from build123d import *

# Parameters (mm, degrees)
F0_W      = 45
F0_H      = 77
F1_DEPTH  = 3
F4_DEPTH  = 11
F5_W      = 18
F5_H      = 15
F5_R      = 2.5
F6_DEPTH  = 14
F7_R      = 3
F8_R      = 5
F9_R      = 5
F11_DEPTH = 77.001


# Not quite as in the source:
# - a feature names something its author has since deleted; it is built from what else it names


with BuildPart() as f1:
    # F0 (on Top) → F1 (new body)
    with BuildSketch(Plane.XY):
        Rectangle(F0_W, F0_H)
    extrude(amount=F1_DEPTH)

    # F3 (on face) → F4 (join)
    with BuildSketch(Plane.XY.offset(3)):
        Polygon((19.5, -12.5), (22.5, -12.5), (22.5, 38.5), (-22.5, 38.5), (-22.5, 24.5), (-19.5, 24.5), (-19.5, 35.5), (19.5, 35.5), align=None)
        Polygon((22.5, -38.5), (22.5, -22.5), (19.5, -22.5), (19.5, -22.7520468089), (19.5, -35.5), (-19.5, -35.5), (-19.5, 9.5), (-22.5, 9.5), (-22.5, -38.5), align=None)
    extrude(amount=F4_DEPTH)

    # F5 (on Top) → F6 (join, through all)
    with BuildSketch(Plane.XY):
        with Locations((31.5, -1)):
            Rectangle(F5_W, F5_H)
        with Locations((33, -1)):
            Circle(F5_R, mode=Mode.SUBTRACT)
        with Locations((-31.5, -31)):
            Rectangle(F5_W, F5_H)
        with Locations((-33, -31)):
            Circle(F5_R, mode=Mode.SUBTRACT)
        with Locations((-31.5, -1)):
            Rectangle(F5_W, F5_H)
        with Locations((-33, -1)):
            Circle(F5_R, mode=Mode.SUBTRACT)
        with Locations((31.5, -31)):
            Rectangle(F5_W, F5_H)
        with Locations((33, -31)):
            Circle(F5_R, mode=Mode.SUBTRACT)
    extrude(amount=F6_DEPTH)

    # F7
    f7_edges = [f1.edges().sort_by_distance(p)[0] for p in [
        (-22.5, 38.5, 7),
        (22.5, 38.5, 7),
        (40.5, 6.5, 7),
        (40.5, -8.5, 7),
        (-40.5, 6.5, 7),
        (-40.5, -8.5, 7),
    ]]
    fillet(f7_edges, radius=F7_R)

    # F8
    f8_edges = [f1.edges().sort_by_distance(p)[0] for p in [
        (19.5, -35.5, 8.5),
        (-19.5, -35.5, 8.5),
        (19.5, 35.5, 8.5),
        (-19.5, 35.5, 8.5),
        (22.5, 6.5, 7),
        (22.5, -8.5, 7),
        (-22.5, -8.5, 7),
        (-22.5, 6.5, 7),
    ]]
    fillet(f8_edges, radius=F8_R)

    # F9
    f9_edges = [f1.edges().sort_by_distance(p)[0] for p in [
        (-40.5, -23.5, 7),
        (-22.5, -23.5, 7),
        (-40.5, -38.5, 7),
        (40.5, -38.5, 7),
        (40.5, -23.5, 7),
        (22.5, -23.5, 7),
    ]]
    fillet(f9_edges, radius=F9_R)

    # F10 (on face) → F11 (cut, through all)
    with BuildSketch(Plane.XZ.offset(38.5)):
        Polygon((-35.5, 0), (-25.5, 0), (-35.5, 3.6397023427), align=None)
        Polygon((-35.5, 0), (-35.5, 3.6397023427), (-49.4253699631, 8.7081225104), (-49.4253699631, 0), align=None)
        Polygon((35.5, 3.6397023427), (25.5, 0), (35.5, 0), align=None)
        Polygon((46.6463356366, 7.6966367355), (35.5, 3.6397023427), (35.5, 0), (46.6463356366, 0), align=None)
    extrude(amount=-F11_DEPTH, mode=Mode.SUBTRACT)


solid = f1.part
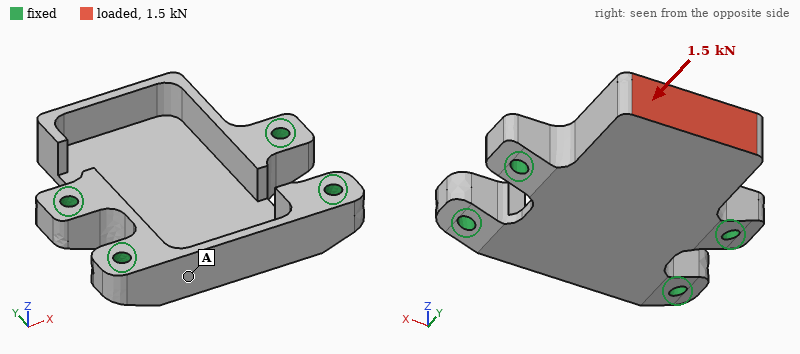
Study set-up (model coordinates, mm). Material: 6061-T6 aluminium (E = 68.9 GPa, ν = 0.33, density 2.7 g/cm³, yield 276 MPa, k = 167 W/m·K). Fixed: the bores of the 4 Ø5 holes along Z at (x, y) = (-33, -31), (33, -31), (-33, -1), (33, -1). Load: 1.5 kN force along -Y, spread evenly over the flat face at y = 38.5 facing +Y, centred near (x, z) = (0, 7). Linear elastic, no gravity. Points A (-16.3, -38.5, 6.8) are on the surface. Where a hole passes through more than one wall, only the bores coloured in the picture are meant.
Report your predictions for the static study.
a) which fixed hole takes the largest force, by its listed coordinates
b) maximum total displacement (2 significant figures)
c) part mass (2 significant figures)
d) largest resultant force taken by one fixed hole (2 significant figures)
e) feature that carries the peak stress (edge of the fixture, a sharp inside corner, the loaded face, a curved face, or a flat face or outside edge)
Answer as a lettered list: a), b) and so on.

a) (33, -1)
b) 0.27 mm
c) 79 g
d) 650 N
e) a curved face
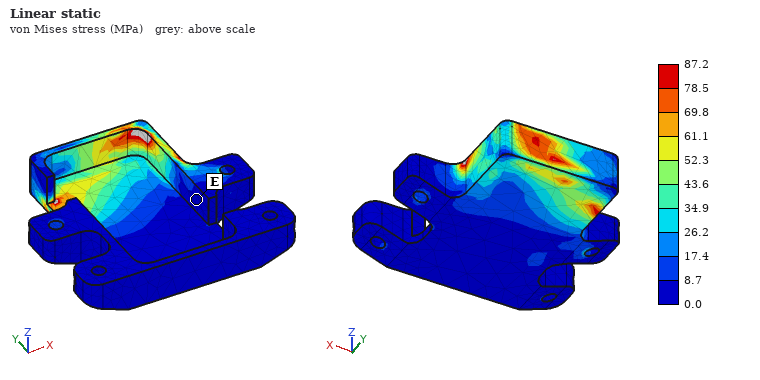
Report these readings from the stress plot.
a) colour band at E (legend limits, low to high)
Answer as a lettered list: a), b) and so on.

a) 0.0 to 8.7 MPa
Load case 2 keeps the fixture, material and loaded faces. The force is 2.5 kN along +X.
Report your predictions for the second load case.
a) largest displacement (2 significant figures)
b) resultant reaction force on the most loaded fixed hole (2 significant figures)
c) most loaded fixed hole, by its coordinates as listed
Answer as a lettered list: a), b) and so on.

a) 0.43 mm
b) 2.0 kN
c) (33, -1)
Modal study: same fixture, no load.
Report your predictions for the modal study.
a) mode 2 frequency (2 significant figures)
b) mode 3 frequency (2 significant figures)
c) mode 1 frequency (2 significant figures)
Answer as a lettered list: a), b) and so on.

a) 4900 Hz
b) 7700 Hz
c) 2100 Hz
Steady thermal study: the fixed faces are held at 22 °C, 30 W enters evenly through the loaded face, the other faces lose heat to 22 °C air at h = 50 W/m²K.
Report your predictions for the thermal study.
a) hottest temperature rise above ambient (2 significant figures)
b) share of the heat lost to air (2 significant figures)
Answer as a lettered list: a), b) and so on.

a) 43 K
b) 22 %
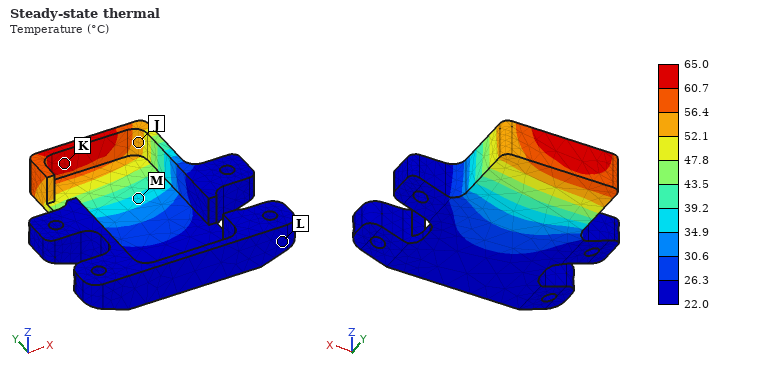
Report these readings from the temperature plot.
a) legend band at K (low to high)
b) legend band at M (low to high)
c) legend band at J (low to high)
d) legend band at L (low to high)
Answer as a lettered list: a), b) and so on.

a) 60.7 to 65.0 °C
b) 34.9 to 39.2 °C
c) 52.1 to 56.4 °C
d) 22.0 to 26.3 °C
